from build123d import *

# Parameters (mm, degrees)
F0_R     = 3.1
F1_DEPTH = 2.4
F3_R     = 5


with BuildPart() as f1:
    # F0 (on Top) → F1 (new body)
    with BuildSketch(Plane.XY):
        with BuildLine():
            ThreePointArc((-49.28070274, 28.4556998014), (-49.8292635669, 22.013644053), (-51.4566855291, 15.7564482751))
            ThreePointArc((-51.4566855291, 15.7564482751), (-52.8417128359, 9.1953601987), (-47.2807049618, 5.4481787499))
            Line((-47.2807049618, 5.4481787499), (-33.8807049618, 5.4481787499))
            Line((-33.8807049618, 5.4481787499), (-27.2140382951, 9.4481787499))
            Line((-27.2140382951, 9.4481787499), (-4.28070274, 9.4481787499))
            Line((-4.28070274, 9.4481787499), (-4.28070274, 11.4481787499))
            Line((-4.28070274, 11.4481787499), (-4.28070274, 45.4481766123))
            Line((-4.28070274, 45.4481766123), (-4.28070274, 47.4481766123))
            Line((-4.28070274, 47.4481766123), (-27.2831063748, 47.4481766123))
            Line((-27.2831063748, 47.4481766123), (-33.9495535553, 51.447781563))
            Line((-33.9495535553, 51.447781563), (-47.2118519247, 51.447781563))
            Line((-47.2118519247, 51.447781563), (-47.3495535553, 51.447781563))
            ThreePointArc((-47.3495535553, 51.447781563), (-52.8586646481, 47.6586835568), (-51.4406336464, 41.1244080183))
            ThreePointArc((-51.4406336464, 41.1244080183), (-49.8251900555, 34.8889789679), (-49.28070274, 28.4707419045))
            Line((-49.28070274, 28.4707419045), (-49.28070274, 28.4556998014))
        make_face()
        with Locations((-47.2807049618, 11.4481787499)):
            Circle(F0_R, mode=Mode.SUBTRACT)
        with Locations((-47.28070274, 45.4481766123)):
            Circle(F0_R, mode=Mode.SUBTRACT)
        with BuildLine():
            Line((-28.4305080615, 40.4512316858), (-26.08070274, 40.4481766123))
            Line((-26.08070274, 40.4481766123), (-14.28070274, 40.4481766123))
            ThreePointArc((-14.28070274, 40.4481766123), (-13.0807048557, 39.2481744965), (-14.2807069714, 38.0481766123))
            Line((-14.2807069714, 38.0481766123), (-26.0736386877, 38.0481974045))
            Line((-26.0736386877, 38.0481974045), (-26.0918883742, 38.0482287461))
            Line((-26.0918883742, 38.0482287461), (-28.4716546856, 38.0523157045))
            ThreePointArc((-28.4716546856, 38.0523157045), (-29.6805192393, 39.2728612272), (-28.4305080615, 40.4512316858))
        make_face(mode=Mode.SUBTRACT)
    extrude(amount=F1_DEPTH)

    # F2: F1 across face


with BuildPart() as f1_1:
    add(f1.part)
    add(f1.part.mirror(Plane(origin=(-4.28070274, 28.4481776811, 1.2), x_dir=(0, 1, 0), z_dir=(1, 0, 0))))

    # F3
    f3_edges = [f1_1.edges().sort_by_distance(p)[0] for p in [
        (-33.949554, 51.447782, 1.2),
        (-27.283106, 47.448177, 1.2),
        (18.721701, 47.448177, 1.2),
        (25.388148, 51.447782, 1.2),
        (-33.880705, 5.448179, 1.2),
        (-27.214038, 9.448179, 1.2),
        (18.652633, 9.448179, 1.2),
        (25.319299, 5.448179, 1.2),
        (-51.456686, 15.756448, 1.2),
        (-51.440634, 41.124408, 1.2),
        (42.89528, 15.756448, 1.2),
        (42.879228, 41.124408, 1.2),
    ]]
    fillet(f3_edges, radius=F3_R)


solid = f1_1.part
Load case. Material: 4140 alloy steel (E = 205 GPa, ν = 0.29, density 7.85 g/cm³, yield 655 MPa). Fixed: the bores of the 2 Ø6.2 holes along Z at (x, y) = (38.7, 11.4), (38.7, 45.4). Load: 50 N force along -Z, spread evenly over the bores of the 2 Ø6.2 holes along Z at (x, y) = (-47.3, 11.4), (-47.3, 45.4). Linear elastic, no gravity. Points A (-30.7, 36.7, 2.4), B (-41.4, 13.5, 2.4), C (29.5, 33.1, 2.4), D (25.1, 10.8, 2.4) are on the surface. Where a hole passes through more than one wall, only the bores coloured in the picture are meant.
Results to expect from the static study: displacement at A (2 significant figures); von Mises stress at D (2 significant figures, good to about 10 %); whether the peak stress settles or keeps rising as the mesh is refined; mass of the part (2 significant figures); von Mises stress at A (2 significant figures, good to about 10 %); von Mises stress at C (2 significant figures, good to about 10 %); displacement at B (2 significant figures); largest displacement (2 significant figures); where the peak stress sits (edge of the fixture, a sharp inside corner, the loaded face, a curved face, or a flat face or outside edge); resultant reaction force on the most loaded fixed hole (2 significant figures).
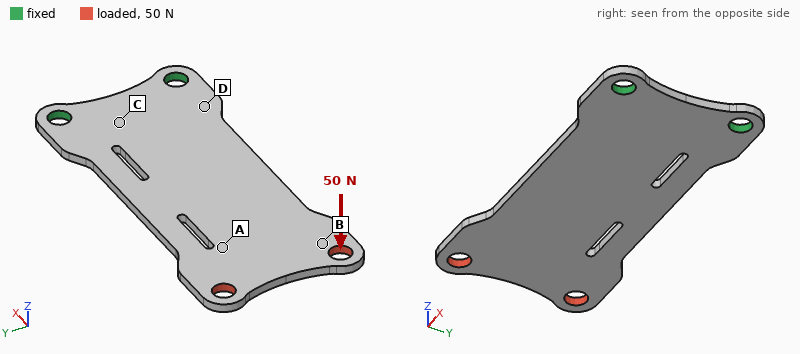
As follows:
0.78 mm
88 MPa
keeps rising
69 g
23 MPa
74 MPa
0.98 mm
1.2 mm
edge of the fixture
25 N
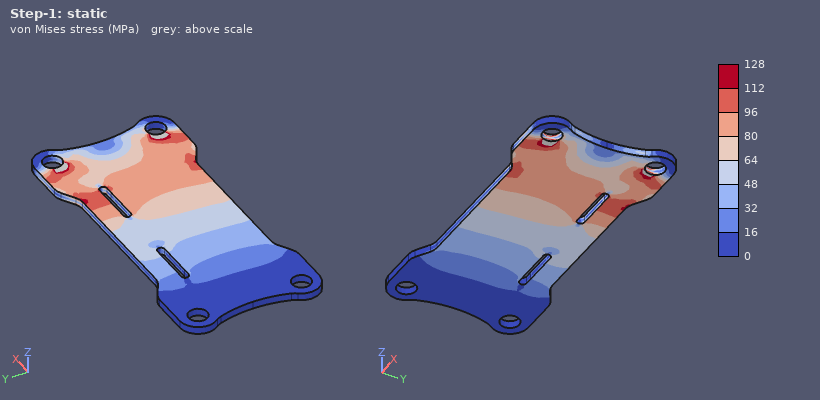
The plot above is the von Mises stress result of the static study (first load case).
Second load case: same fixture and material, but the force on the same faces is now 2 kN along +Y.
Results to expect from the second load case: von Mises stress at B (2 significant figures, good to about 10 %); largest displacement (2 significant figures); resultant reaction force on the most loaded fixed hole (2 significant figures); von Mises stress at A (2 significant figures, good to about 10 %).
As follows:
44 MPa
0.21 mm
5.0 kN
39 MPa
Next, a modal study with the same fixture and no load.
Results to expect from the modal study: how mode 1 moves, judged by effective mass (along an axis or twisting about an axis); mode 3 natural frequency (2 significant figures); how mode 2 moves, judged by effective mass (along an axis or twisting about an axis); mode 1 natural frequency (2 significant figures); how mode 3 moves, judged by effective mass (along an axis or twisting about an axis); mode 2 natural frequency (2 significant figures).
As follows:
along Z
1600 Hz
twisting about X
250 Hz
along Z
1100 Hz
